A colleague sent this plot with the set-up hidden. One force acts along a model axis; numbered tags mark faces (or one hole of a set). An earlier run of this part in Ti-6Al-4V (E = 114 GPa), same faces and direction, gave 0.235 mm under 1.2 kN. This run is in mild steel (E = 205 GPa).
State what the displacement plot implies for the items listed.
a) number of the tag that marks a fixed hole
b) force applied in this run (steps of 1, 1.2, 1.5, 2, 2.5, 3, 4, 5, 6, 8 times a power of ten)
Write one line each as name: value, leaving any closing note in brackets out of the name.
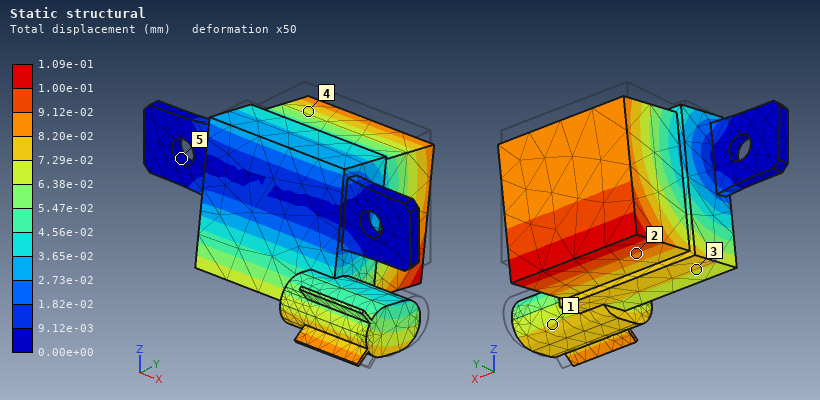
number of the tag that marks a fixed hole: 5
force applied in this run: 1 kN
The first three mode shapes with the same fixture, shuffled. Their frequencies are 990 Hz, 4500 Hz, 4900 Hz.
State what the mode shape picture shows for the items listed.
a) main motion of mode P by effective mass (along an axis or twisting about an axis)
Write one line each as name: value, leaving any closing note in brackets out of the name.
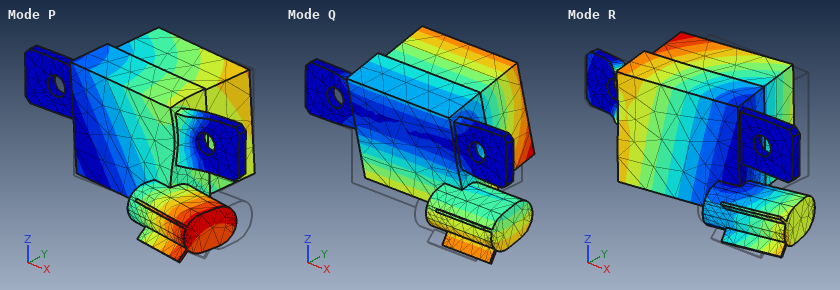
main motion of mode P by effective mass: along Y
